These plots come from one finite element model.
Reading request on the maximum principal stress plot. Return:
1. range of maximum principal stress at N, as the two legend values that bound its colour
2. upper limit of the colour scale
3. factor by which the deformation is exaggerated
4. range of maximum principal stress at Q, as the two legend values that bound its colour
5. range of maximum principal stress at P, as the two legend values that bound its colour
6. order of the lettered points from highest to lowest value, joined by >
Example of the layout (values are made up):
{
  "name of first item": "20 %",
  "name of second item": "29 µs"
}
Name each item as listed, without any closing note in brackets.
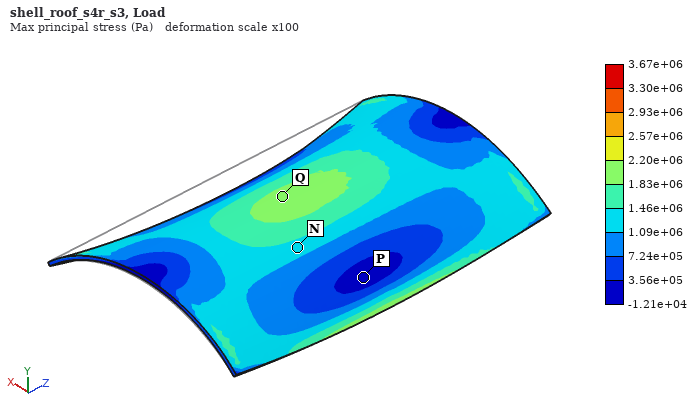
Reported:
{
  "range of maximum principal stress at N, as the two legend values that bound its colour": "1.09e+06 to 1.46e+06 Pa",
  "upper limit of the colour scale": "3.67e+06 Pa",
  "factor by which the deformation is exaggerated": "100",
  "range of maximum principal stress at Q, as the two legend values that bound its colour": "1.83e+06 to 2.20e+06 Pa",
  "range of maximum principal stress at P, as the two legend values that bound its colour": "-1.21e+04 to 3.56e+05 Pa",
  "order of the lettered points from highest to lowest value, joined by >": "Q > N > P"
}
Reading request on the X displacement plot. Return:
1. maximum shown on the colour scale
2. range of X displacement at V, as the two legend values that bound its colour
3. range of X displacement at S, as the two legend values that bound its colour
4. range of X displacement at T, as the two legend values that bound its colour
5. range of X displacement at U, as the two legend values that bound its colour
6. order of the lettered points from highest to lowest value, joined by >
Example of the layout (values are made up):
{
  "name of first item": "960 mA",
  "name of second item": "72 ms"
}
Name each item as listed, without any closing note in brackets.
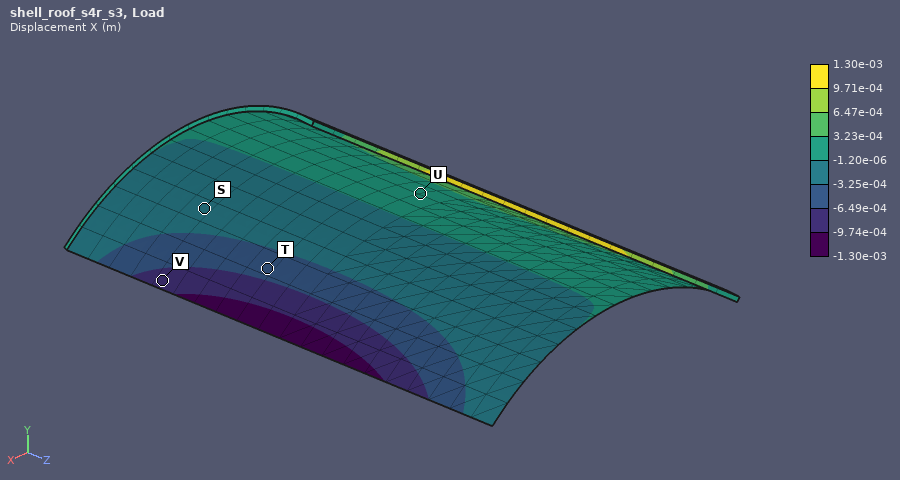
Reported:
{
  "maximum shown on the colour scale": "1.30e-03 m",
  "range of X displacement at V, as the two legend values that bound its colour": "-9.74e-04 to -6.49e-04 m",
  "range of X displacement at S, as the two legend values that bound its colour": "-3.25e-04 to -1.20e-06 m",
  "range of X displacement at T, as the two legend values that bound its colour": "-6.49e-04 to -3.25e-04 m",
  "range of X displacement at U, as the two legend values that bound its colour": "-1.20e-06 to 3.23e-04 m",
  "order of the lettered points from highest to lowest value, joined by >": "U > S > T > V"
}
